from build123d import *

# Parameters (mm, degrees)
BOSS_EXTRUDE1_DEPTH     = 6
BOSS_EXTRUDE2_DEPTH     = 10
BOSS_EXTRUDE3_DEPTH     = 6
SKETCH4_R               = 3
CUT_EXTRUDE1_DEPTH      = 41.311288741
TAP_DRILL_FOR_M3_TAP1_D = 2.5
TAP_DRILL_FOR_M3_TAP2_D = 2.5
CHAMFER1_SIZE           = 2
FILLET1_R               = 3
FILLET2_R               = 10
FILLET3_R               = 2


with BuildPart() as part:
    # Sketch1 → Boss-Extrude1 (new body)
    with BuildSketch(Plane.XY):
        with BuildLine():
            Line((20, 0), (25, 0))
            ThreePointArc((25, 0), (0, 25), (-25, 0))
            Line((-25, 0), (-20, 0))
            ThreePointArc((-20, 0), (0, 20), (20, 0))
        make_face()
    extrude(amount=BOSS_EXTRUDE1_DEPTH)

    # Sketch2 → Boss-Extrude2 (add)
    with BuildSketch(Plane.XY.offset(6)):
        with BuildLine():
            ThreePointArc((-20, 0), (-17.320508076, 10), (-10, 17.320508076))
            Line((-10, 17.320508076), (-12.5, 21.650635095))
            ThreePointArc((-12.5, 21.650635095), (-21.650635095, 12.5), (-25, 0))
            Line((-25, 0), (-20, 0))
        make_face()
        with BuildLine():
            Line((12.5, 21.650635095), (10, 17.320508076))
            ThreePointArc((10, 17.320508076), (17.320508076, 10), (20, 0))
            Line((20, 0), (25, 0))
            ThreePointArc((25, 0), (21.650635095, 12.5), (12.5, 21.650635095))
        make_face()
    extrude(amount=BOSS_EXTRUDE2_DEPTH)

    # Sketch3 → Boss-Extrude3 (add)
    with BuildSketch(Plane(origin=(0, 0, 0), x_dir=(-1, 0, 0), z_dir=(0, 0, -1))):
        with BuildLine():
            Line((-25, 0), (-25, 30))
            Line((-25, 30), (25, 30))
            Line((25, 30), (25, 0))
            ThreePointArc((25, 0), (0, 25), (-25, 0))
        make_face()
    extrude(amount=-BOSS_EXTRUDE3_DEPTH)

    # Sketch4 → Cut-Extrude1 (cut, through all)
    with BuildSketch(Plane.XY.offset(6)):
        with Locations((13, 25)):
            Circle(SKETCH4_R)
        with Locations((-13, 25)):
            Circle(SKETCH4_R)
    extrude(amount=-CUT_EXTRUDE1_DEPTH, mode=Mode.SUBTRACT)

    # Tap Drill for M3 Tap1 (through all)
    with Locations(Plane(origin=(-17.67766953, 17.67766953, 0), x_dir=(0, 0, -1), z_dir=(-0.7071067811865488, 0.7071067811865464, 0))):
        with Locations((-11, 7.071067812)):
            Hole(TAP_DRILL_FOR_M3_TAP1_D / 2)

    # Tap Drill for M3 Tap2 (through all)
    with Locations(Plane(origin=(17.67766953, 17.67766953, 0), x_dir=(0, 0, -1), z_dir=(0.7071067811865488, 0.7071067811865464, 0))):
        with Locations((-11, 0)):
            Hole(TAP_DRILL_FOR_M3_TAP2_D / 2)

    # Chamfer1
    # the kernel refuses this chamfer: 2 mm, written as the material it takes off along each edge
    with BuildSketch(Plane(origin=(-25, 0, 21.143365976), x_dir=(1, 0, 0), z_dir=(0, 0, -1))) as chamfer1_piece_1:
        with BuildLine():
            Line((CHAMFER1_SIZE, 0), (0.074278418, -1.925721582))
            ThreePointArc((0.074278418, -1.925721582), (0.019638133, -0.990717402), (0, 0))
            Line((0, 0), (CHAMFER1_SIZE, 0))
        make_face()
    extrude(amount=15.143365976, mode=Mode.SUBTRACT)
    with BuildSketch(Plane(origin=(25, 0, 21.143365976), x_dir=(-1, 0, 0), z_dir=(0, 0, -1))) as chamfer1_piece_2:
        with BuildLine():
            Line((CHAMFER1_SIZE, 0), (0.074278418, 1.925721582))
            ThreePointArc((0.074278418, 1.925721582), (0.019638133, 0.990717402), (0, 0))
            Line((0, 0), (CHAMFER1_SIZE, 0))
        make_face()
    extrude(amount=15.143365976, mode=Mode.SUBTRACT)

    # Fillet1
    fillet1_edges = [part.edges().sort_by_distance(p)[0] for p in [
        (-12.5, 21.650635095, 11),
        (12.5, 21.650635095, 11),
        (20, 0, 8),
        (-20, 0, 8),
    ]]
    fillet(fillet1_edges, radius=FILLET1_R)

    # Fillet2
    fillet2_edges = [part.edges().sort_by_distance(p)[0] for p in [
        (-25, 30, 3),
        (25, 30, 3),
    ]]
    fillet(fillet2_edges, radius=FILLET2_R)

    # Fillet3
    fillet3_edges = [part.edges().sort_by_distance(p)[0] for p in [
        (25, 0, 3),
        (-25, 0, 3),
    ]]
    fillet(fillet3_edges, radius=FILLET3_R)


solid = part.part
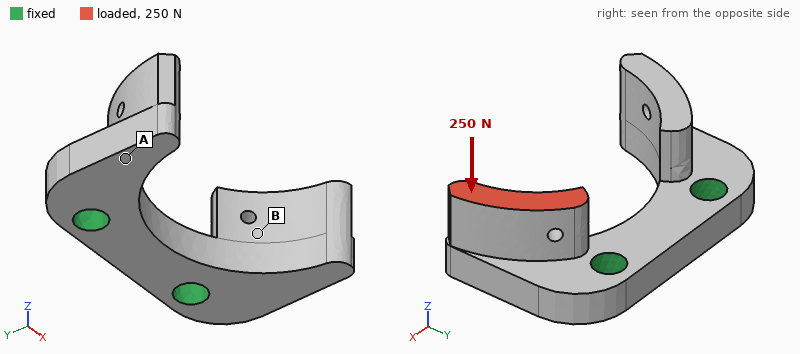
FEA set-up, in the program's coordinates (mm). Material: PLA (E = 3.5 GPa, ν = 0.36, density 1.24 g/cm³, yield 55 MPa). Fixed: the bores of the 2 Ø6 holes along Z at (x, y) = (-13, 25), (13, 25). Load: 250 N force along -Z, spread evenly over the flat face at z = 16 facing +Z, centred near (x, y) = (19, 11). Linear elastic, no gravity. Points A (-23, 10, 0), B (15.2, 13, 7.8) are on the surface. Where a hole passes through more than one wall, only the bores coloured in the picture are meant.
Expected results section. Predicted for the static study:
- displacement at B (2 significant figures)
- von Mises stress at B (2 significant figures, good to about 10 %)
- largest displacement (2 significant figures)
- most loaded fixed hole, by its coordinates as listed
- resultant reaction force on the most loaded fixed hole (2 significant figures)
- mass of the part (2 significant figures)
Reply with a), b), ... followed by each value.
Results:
a) 0.20 mm
b) 11 MPa
c) 0.63 mm
d) (13, 25)
e) 260 N
f) 8.4 g
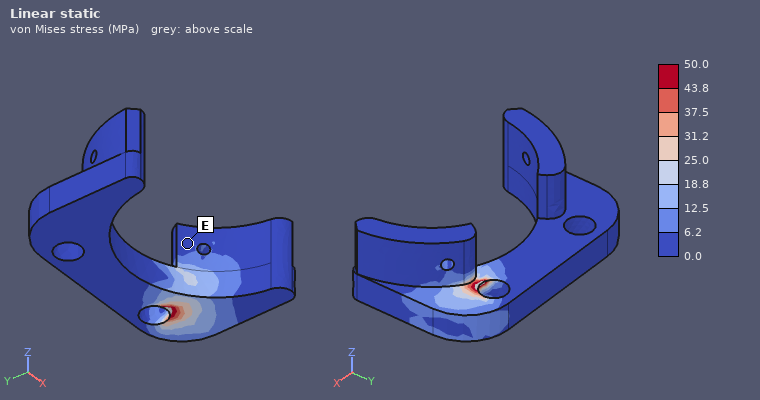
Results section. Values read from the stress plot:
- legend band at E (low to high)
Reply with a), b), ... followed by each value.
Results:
a) 0.0 to 6.2 MPa
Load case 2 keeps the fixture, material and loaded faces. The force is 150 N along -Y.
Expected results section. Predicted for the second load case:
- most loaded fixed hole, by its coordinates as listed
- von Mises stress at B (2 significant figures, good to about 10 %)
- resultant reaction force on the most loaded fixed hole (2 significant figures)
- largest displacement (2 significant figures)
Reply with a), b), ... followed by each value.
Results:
a) (13, 25)
b) 12 MPa
c) 160 N
d) 0.55 mm
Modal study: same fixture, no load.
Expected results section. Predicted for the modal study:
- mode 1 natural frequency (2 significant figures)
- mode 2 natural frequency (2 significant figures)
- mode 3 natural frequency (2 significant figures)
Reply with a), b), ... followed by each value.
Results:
a) 2400 Hz
b) 2500 Hz
c) 3500 Hz
